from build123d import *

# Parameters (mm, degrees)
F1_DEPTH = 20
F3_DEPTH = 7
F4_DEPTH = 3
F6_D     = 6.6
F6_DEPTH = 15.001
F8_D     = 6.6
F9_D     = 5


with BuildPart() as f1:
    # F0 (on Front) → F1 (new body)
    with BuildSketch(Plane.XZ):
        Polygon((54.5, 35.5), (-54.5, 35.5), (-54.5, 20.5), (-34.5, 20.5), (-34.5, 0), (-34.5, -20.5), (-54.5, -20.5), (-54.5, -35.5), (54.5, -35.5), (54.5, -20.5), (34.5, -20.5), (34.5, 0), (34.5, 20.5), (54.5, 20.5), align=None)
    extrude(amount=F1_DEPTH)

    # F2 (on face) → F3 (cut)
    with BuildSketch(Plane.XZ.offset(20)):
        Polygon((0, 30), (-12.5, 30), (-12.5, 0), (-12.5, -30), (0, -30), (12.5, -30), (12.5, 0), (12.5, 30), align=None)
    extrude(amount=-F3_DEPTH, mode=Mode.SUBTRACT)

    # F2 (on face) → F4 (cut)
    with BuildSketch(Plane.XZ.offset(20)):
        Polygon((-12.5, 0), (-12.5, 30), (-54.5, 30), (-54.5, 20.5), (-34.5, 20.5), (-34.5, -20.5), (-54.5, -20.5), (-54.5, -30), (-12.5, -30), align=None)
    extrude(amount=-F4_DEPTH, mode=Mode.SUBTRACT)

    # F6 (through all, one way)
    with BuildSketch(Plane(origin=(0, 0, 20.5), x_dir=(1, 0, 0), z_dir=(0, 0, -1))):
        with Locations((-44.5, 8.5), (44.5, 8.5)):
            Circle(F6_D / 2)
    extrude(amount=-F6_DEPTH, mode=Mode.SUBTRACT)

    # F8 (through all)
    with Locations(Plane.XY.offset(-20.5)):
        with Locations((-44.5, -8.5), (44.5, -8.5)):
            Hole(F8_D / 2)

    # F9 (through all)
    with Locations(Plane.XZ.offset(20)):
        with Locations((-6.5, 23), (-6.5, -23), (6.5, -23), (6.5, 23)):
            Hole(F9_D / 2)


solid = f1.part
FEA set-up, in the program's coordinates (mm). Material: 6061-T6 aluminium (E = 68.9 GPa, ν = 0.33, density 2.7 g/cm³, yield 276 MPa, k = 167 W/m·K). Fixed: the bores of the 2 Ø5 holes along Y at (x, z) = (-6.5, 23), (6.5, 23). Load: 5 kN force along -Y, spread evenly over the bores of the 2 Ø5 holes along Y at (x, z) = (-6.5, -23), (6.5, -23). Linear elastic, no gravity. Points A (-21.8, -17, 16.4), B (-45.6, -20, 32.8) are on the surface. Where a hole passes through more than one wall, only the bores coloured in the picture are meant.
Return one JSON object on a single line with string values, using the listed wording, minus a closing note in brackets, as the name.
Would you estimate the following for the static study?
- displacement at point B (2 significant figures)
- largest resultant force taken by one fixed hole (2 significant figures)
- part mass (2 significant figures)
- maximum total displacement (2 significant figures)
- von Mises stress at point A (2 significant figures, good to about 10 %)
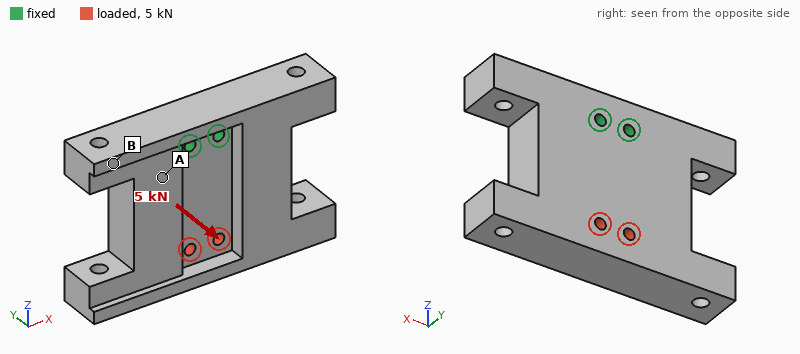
{"displacement at point B": "0.053 mm", "largest resultant force taken by one fixed hole": "2.6 kN", "part mass": "280 g", "maximum total displacement": "0.27 mm", "von Mises stress at point A": "47 MPa"}
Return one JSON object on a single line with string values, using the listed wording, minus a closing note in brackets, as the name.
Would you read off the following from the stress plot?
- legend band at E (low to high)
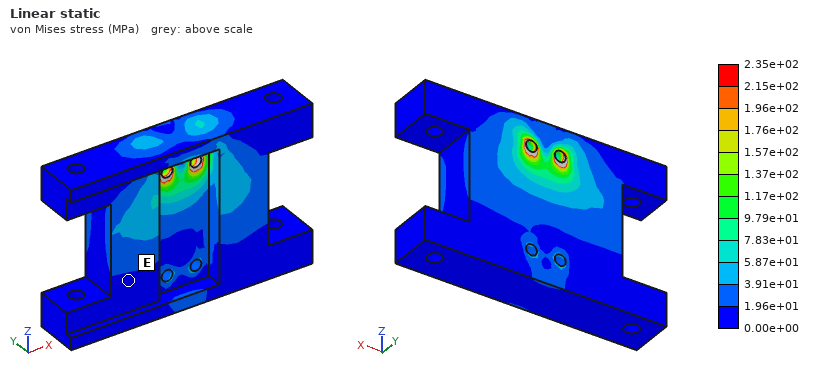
{"legend band at E": "0.00e+00 to 1.96e+01 MPa"}
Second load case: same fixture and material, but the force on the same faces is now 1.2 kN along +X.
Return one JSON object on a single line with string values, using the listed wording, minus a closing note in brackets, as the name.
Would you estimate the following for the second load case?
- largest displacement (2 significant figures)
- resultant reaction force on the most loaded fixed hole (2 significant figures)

{"largest displacement": "30 µm", "resultant reaction force on the most loaded fixed hole": "3.2 kN"}
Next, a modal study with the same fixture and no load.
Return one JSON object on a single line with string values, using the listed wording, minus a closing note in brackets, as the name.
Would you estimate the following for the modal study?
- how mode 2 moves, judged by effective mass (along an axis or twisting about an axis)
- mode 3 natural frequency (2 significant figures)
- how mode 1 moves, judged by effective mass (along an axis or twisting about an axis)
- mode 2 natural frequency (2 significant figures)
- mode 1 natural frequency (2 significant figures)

{"how mode 2 moves, judged by effective mass": "along X", "mode 3 natural frequency": "2900 Hz", "how mode 1 moves, judged by effective mass": "along Y", "mode 2 natural frequency": "2700 Hz", "mode 1 natural frequency": "2100 Hz"}
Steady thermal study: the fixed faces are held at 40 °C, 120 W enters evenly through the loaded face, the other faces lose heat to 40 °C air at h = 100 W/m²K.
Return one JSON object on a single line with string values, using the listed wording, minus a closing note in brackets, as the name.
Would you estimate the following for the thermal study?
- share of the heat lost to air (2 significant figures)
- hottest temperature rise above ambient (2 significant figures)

{"share of the heat lost to air": "29 %", "hottest temperature rise above ambient": "38 K"}
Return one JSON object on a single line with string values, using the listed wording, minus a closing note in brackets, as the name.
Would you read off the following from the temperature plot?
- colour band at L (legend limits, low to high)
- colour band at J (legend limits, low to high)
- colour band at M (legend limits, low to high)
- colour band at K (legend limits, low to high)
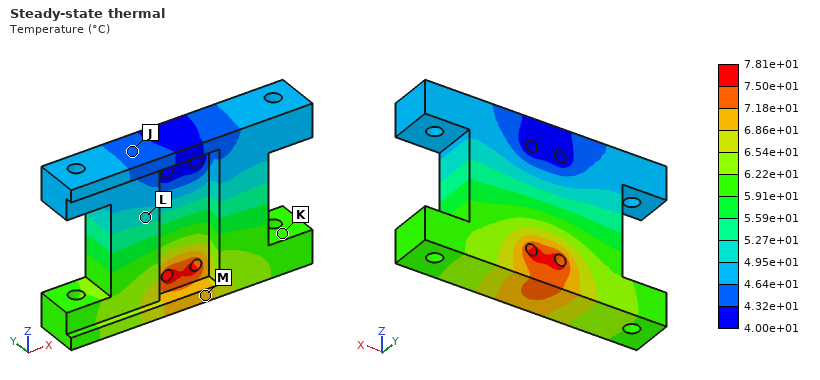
{"colour band at L": "4.95e+01 to 5.27e+01 °C", "colour band at J": "4.32e+01 to 4.64e+01 °C", "colour band at M": "6.86e+01 to 7.18e+01 °C", "colour band at K": "5.91e+01 to 6.22e+01 °C"}
